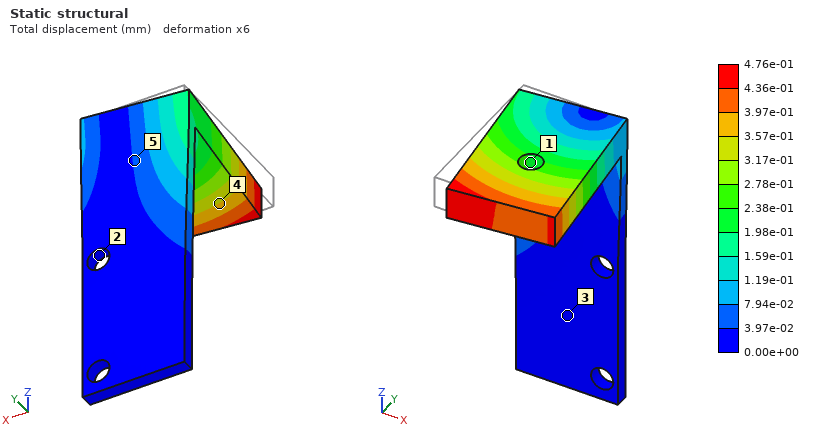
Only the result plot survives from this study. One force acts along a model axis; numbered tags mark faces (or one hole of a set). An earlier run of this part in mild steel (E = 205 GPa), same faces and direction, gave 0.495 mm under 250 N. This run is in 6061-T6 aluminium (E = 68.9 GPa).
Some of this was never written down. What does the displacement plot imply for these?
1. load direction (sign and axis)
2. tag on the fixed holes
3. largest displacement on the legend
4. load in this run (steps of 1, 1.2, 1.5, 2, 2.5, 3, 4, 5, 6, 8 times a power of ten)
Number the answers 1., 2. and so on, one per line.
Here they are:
1. +X
2. 2
3. 4.76e-01 mm
4. 80 N
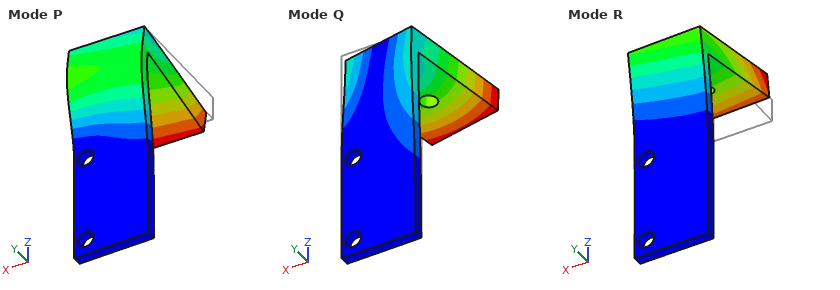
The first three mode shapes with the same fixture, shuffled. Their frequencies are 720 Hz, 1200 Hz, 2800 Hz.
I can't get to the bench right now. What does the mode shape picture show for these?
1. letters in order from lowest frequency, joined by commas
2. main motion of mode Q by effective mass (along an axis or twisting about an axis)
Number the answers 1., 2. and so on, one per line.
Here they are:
1. R, Q, P
2. along X
